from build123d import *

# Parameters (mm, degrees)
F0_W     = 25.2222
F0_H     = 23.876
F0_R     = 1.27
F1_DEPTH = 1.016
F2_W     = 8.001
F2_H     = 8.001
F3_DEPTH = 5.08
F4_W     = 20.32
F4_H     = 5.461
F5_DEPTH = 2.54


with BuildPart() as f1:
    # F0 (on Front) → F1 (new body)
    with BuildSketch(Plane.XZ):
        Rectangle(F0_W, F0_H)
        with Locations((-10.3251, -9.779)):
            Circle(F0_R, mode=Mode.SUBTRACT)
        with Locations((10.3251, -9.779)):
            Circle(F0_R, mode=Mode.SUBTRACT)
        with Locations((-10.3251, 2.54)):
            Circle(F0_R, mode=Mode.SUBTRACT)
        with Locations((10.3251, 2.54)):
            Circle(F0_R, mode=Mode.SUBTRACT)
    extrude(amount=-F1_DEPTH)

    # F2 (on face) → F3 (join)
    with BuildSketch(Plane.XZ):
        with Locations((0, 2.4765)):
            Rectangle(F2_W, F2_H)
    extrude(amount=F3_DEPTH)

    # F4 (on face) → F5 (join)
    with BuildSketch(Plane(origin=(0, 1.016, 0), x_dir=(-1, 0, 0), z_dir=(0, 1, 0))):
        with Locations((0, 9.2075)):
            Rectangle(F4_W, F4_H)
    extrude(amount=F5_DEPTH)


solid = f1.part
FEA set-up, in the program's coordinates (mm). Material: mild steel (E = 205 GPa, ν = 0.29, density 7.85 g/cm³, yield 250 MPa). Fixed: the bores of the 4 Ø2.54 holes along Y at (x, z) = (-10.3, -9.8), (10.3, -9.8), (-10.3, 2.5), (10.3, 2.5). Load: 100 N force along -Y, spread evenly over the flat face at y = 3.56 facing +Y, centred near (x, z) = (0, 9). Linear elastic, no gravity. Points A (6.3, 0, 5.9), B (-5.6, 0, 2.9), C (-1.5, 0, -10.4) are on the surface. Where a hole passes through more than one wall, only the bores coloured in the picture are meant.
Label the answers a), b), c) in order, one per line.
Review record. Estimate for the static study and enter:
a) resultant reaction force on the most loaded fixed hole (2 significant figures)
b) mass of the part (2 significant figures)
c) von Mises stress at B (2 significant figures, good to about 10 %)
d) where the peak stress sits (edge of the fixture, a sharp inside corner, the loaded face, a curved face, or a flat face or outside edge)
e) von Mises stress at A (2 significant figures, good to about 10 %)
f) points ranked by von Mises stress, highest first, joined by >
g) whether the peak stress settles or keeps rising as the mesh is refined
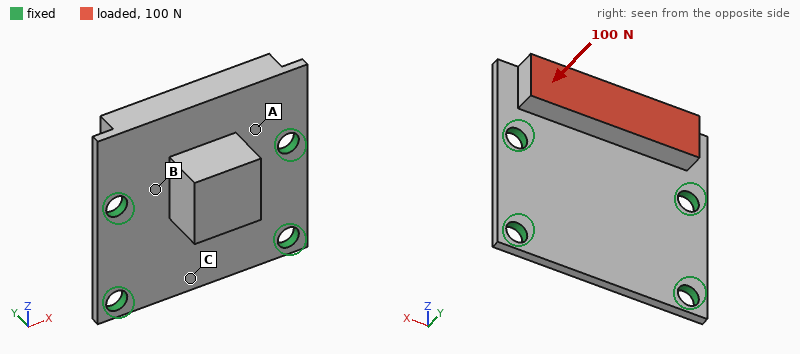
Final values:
a) 60 N
b) 9.4 g
c) 23 MPa
d) edge of the fixture
e) 47 MPa
f) A > B > C
g) keeps rising
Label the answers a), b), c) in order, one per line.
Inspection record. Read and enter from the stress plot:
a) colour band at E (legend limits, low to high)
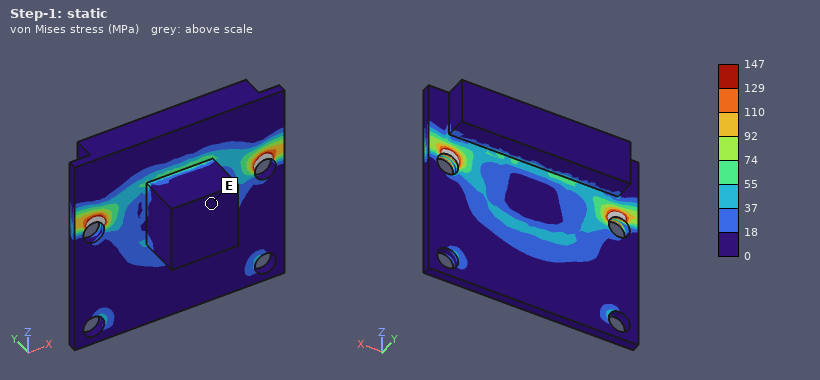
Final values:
a) 0 to 18 MPa
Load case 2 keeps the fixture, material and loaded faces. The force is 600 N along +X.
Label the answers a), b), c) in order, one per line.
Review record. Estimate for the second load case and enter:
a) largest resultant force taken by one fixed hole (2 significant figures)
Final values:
a) 340 N
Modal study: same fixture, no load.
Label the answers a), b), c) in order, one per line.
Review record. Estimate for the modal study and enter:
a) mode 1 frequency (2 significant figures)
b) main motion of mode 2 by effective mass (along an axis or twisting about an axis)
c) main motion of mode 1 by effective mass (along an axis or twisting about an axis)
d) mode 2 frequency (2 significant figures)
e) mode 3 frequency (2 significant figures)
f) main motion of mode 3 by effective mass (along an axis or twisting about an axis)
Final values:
a) 6300 Hz
b) along Y
c) along Y
d) 12 kHz
e) 19 kHz
f) twisting about Z
